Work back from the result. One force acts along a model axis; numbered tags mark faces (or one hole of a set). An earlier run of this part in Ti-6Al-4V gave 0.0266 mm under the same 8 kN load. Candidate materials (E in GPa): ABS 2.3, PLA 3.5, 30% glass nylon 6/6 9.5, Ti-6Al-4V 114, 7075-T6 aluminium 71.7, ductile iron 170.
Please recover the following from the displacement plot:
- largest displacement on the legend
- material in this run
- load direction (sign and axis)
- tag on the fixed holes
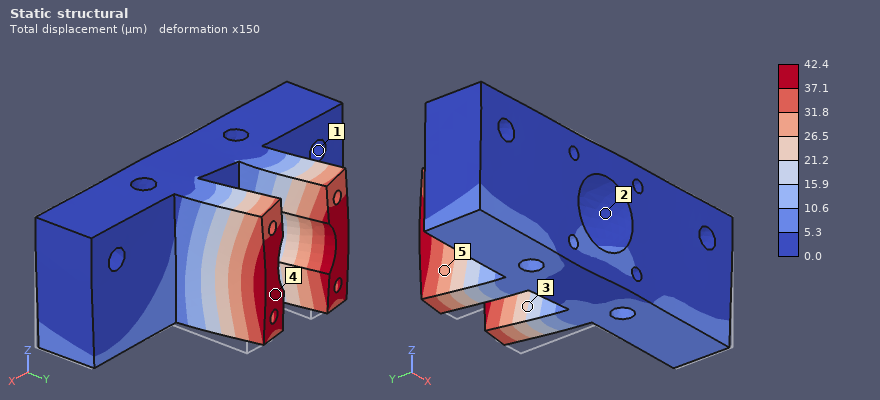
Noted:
42.4 µm
7075-T6 aluminium
-X
1
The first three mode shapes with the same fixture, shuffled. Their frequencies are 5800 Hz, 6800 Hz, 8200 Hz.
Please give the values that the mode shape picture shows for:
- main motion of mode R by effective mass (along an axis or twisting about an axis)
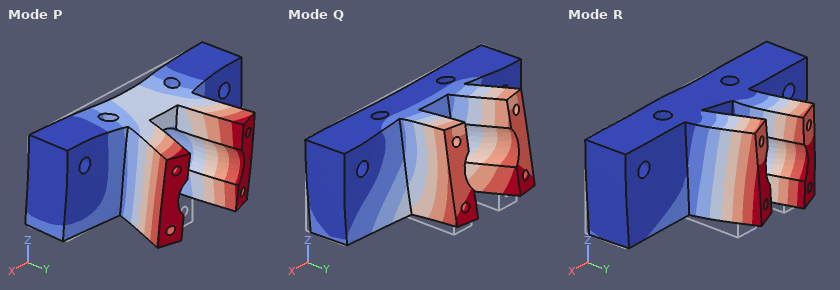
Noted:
along X
